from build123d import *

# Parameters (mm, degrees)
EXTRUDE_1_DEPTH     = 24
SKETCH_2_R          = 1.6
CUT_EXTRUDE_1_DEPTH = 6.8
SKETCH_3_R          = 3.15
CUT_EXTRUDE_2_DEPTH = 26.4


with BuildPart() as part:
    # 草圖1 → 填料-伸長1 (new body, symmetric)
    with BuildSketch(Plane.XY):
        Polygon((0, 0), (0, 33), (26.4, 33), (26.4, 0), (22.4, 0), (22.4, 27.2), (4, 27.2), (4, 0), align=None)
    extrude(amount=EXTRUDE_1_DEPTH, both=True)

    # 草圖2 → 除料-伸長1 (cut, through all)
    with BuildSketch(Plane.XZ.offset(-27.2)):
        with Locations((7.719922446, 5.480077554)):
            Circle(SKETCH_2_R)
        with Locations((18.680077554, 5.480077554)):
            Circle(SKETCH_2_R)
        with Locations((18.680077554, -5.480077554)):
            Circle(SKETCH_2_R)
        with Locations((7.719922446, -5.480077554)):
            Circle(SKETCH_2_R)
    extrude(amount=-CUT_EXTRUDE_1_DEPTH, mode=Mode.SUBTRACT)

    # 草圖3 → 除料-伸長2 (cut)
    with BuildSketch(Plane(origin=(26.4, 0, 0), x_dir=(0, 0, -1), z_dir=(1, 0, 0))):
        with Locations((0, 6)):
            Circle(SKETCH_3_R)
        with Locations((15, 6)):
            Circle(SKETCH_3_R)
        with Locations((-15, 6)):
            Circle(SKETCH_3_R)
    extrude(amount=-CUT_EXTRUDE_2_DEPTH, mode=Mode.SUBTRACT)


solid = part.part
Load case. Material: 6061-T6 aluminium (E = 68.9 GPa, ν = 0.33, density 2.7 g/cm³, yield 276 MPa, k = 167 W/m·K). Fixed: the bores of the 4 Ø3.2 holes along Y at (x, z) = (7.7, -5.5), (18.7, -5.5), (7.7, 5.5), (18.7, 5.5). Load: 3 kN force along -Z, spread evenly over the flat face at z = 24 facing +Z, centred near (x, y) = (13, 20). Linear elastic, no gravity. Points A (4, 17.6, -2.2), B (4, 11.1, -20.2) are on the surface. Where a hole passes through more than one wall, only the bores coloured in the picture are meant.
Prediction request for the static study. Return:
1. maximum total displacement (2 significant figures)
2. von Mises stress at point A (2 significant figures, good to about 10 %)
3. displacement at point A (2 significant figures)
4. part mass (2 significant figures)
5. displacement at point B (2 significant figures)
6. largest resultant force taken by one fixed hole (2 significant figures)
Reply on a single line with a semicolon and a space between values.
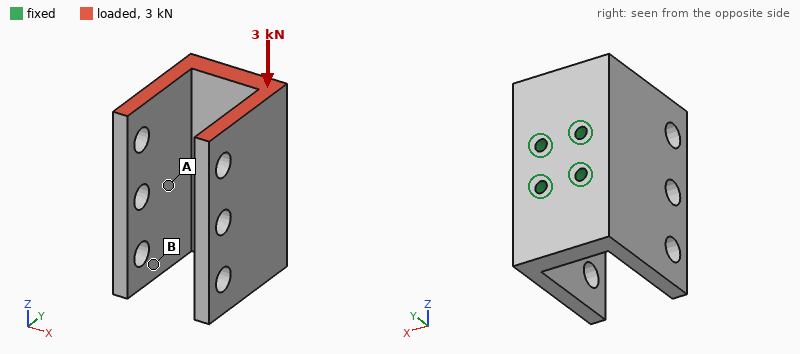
40 µm; 14 MPa; 13 µm; 46 g; 25 µm; 1.3 kN
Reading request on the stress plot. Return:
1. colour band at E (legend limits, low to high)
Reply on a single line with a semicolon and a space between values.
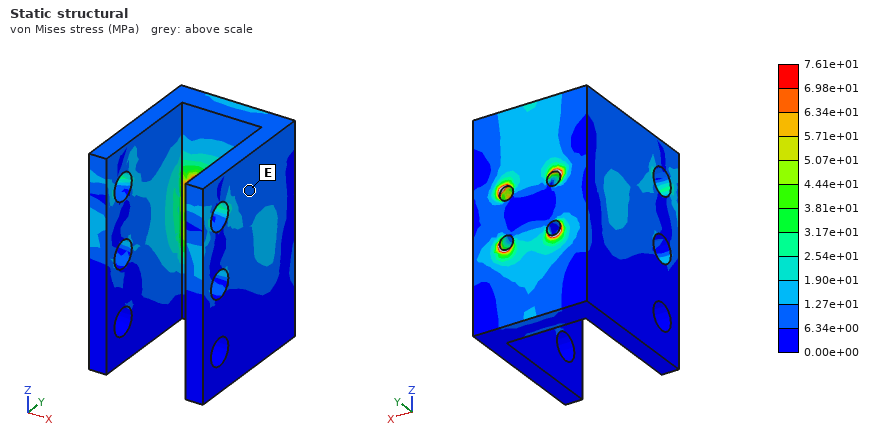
6.34e+00 to 1.27e+01 MPa
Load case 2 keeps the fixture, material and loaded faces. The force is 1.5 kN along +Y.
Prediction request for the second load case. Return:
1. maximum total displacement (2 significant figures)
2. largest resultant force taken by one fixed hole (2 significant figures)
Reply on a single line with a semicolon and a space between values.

46 µm; 1.4 kN
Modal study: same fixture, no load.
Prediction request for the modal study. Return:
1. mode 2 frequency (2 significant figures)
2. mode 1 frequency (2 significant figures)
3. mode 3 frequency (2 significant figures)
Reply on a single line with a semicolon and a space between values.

3700 Hz; 3700 Hz; 5600 Hz
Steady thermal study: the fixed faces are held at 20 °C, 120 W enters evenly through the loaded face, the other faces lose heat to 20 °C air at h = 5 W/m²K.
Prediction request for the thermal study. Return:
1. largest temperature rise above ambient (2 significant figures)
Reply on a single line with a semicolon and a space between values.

69 K
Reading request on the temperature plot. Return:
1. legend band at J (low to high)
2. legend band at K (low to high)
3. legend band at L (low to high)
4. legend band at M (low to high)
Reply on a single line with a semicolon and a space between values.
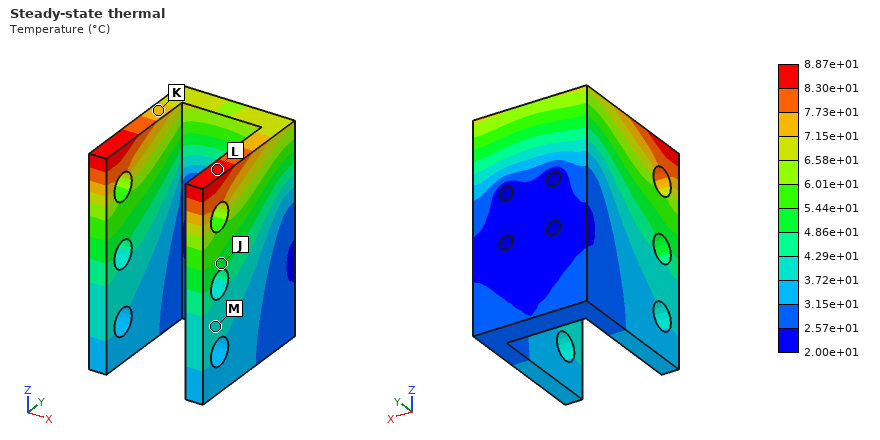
4.86e+01 to 5.44e+01 °C; 7.15e+01 to 7.73e+01 °C; 8.30e+01 to 8.87e+01 °C; 3.72e+01 to 4.29e+01 °C
